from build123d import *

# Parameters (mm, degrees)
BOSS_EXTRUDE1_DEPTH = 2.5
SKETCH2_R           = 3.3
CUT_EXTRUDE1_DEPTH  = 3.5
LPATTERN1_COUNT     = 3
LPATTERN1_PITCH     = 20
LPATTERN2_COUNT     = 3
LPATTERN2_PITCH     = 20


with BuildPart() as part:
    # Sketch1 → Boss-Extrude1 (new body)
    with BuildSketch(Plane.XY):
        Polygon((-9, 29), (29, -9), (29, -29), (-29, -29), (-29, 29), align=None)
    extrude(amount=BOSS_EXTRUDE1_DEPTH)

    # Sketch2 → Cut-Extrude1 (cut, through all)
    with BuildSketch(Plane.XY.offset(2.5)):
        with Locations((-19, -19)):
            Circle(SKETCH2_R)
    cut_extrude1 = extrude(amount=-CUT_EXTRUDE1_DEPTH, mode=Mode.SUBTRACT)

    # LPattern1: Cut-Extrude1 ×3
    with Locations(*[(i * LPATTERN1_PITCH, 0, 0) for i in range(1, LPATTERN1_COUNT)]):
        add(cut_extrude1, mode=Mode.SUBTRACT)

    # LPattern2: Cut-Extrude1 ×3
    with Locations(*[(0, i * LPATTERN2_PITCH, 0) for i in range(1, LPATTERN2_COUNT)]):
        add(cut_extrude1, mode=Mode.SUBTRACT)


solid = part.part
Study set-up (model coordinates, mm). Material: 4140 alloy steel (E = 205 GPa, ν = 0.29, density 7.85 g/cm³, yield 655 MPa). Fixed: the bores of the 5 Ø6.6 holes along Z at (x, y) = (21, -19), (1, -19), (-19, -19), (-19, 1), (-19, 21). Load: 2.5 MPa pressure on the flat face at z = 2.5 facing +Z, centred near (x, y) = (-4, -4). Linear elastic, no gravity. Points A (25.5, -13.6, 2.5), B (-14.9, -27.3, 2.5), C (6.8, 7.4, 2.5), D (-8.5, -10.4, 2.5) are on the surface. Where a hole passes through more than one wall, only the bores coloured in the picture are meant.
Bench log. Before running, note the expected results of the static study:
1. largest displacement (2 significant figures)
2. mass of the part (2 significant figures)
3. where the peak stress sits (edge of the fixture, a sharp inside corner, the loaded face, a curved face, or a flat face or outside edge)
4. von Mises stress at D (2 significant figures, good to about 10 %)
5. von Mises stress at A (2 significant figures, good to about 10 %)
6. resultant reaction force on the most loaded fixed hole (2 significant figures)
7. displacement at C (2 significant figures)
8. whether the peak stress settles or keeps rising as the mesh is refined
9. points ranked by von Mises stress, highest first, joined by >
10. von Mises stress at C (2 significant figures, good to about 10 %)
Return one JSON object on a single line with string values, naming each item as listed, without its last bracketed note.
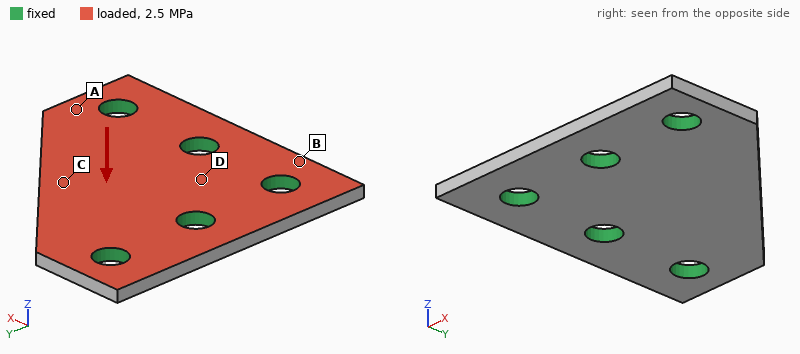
{"largest displacement": "0.18 mm", "mass of the part": "48 g", "where the peak stress sits": "edge of the fixture", "von Mises stress at D": "100 MPa", "von Mises stress at A": "210 MPa", "resultant reaction force on the most loaded fixed hole": "1.4 kN", "displacement at C": "0.15 mm", "whether the peak stress settles or keeps rising as the mesh is refined": "keeps rising", "points ranked by von Mises stress, highest first, joined by >": "A > C > D > B", "von Mises stress at C": "160 MPa"}
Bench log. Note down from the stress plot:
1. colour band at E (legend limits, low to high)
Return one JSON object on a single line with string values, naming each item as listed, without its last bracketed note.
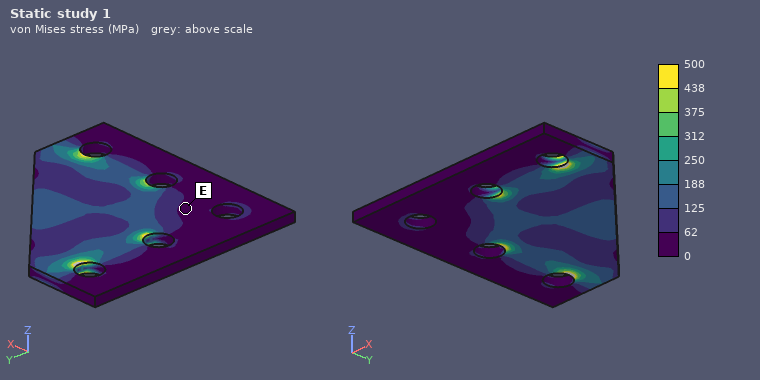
{"colour band at E": "0 to 62 MPa"}
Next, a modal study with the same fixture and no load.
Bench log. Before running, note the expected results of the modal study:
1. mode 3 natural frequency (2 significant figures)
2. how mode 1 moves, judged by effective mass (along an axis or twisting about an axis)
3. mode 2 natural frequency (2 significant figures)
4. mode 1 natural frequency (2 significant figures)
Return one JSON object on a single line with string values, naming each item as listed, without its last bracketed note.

{"mode 3 natural frequency": "17 kHz", "how mode 1 moves, judged by effective mass": "along Z", "mode 2 natural frequency": "12 kHz", "mode 1 natural frequency": "5800 Hz"}
